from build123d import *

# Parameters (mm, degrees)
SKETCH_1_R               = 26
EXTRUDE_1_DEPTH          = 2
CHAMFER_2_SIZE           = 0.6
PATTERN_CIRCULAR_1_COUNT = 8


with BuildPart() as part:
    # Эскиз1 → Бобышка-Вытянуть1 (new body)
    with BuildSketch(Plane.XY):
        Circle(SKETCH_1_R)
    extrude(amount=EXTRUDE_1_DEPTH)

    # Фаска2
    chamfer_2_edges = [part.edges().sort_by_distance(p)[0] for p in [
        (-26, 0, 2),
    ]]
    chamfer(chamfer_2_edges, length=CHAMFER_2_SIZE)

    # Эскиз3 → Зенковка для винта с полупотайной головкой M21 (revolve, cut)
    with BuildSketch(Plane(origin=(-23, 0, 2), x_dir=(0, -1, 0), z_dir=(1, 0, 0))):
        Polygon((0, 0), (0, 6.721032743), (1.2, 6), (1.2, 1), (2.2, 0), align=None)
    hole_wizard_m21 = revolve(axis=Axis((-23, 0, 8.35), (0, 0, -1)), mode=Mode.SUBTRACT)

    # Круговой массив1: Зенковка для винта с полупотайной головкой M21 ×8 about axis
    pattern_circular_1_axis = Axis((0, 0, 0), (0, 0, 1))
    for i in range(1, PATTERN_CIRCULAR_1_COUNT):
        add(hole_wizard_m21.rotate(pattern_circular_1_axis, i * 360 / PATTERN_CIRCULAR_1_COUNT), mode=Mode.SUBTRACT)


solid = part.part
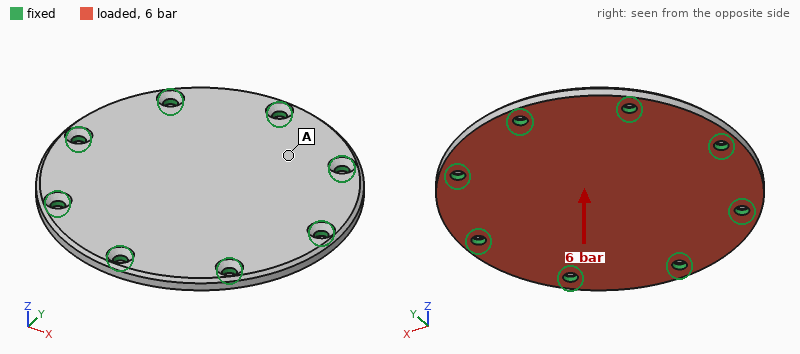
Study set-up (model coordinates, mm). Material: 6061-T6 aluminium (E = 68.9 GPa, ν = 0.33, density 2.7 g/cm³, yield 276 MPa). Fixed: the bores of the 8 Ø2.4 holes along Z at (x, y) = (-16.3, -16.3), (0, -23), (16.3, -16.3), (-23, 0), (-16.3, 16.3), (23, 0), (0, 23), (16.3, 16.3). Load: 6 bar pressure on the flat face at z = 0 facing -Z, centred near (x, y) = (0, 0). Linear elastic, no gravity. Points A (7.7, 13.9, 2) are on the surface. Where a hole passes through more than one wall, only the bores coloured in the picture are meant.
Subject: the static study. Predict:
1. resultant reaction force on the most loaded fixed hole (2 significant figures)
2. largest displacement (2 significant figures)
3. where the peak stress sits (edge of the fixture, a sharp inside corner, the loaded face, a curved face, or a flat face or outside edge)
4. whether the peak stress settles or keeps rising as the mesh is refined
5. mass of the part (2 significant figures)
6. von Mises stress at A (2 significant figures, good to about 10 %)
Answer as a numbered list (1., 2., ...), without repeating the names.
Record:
1. 200 N
2. 77 µm
3. edge of the fixture
4. keeps rising
5. 11 g
6. 29 MPa
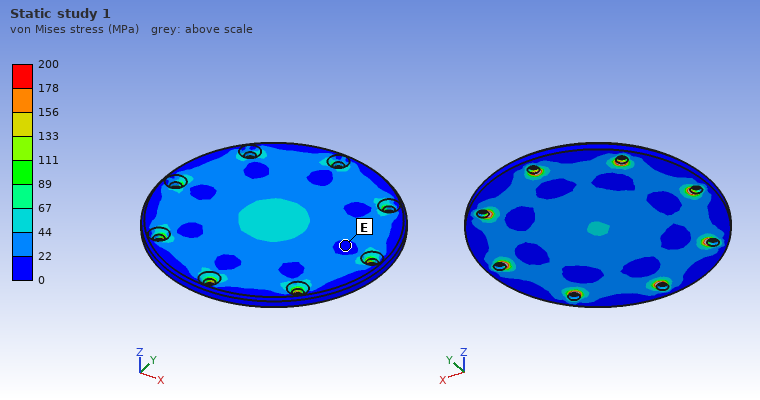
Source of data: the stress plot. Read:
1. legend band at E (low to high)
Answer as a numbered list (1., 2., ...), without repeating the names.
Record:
1. 0 to 22 MPa
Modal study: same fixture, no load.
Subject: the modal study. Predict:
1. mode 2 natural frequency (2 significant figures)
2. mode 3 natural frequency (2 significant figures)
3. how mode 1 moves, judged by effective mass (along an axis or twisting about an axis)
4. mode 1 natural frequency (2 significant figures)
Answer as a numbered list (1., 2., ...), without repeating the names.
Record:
1. 16 kHz
2. 16 kHz
3. along Z
4. 7500 Hz
